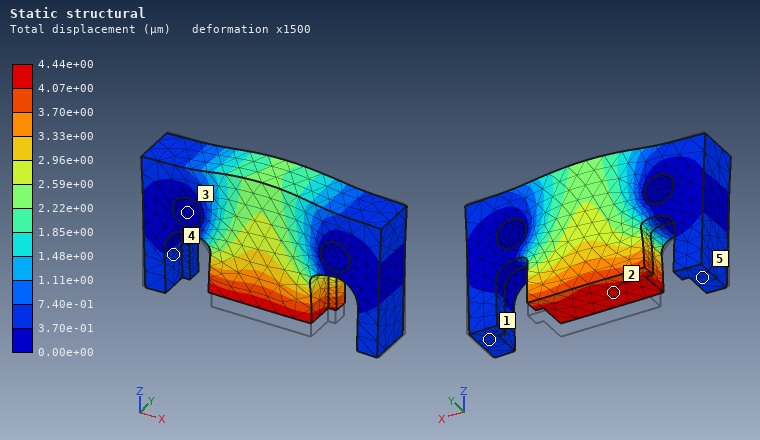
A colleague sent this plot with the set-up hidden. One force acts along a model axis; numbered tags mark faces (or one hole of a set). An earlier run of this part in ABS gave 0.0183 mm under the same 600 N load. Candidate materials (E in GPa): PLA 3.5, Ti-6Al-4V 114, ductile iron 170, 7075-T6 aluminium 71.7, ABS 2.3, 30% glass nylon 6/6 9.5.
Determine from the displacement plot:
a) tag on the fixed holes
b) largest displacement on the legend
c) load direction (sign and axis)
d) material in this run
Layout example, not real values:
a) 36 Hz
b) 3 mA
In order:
a) 3
b) 4.44e+00 µm
c) +Z
d) 30% glass nylon 6/6
